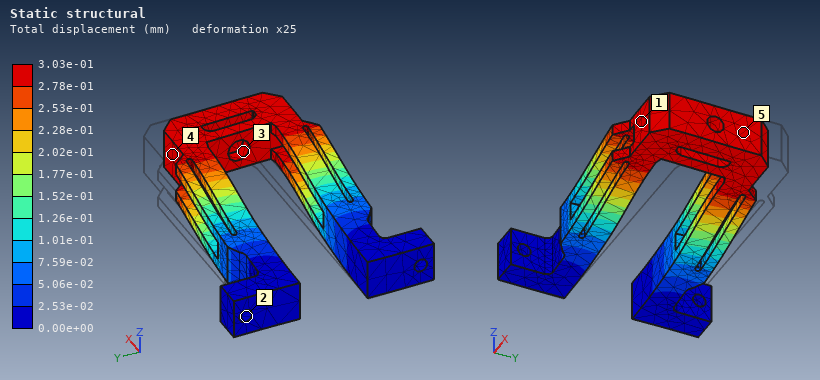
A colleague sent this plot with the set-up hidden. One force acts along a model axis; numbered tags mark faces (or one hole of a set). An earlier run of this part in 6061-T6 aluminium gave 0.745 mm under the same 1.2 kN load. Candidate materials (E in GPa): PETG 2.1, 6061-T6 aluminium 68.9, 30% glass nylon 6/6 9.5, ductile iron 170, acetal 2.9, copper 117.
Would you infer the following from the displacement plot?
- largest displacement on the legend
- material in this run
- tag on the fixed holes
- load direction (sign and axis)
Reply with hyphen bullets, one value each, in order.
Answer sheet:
- 3.03e-01 mm
- ductile iron
- 2
- -Y
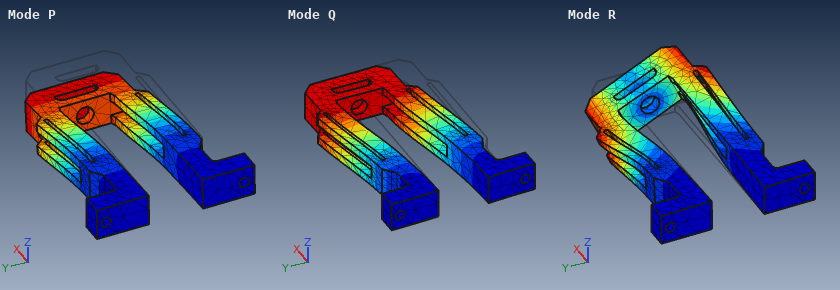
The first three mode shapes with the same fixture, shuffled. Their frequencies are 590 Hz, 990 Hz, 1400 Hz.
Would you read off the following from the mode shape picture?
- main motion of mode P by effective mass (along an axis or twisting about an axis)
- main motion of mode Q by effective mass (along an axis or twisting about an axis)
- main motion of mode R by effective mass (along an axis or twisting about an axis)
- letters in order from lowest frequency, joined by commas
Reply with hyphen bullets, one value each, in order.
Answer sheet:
- along Z
- along Y
- twisting about X
- P, Q, R
